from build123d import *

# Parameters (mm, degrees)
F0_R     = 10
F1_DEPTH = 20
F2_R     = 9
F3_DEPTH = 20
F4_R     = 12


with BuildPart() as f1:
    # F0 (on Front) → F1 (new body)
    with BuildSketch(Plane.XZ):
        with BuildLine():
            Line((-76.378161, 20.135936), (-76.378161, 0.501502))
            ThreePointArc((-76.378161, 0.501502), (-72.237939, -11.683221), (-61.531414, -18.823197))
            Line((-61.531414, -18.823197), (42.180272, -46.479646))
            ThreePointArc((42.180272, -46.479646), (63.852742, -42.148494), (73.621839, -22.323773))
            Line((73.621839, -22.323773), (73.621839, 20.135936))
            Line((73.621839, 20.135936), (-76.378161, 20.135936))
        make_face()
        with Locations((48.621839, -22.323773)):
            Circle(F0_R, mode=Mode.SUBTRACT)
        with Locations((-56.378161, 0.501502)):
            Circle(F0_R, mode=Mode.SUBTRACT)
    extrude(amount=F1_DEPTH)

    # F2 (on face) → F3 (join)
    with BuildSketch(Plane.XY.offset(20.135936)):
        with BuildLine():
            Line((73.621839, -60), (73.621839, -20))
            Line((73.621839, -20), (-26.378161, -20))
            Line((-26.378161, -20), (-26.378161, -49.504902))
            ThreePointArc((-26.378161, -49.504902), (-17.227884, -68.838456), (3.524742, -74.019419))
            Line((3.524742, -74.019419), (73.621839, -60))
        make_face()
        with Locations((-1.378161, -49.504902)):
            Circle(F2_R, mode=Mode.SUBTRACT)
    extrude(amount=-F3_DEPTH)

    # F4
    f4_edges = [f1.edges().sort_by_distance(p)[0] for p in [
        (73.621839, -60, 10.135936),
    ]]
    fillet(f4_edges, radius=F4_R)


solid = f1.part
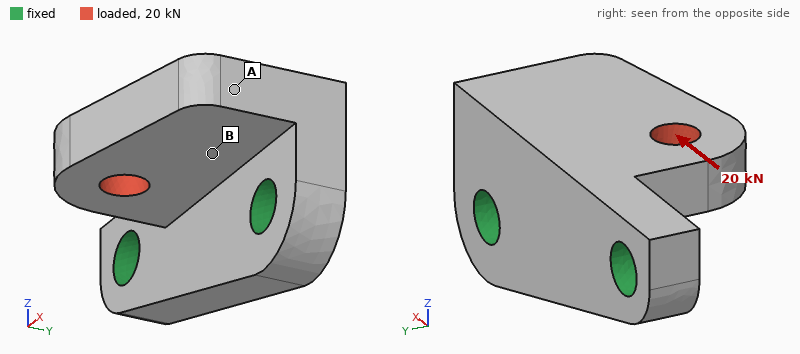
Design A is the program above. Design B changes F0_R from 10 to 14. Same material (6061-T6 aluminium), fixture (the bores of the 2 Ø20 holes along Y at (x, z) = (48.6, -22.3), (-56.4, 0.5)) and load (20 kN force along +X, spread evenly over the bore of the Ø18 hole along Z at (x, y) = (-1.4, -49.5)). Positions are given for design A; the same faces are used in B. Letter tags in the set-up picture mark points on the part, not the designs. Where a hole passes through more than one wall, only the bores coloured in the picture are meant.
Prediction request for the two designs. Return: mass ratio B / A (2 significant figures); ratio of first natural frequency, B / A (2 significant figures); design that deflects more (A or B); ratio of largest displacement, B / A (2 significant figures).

0.95
1.1
A
0.81
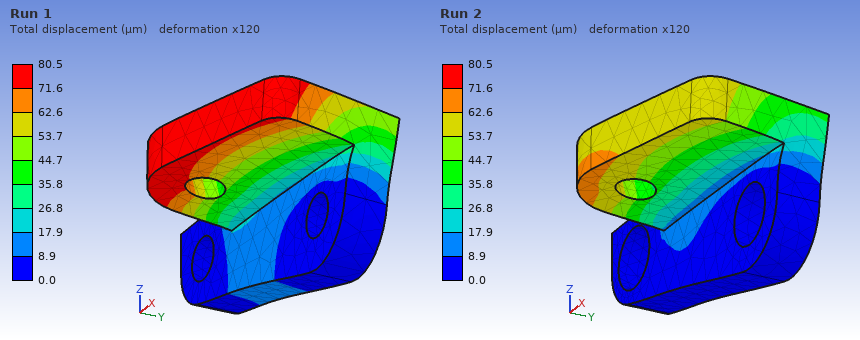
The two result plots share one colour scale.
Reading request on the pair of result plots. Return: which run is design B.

Run 2
